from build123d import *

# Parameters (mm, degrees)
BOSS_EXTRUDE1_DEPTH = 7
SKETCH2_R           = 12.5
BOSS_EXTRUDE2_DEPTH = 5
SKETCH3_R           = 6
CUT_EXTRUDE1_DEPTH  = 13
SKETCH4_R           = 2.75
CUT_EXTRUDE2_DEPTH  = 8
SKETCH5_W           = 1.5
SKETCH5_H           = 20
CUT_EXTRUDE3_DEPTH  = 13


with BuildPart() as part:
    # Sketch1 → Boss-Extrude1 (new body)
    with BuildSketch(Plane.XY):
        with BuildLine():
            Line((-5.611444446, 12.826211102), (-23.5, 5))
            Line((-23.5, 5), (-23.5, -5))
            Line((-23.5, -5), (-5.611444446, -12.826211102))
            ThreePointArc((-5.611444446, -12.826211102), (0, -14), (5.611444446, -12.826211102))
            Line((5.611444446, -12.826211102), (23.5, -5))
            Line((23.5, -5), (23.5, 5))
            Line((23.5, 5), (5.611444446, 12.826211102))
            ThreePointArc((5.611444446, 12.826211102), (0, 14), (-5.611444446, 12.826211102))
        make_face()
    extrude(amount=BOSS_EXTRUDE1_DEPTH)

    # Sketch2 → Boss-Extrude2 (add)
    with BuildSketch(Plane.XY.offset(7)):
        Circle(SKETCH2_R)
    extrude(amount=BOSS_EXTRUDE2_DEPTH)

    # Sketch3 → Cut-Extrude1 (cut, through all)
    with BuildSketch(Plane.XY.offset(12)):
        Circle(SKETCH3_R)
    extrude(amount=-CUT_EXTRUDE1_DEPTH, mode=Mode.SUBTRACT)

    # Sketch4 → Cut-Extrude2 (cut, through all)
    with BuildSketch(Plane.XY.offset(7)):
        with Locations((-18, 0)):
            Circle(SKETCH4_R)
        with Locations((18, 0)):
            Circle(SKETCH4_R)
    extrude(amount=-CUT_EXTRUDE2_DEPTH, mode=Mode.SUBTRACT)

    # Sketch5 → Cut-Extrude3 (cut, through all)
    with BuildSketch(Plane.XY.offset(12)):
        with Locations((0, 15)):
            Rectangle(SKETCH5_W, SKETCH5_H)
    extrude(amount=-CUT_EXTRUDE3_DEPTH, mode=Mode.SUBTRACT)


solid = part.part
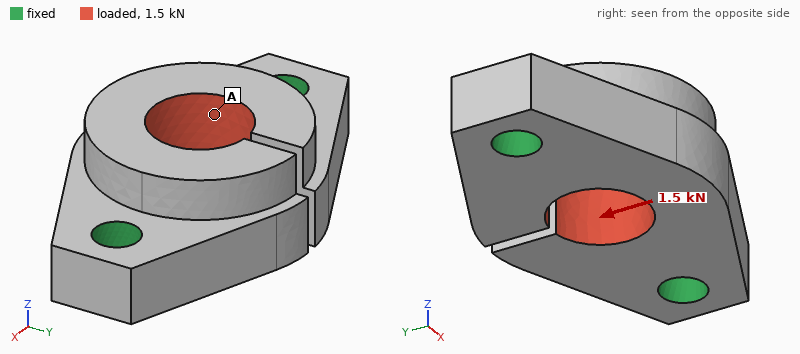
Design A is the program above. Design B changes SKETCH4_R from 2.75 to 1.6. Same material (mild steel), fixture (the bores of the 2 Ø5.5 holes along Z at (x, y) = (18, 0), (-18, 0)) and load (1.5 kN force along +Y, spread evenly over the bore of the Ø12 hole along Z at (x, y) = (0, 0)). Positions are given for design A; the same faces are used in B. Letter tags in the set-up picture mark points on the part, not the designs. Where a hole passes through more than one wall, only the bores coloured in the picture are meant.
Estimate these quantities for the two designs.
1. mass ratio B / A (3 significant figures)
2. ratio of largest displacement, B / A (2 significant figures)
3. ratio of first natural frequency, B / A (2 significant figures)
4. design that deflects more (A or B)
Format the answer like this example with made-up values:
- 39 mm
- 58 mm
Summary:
- 1.03
- 1.4
- 0.85
- B
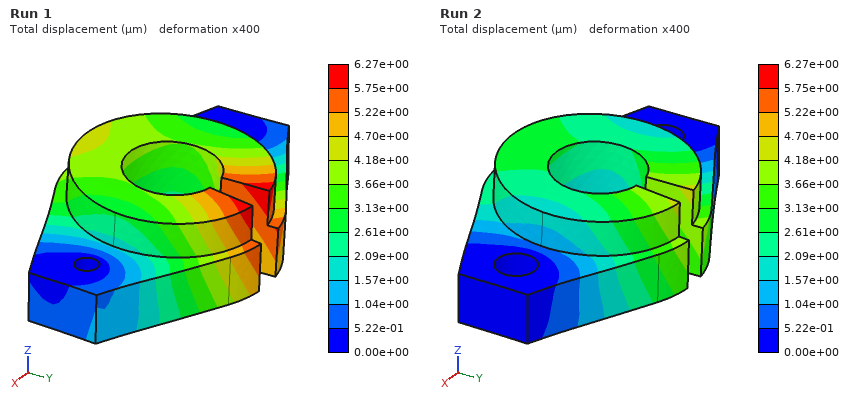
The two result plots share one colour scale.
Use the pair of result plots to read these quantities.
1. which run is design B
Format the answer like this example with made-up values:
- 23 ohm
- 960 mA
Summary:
- Run 1
